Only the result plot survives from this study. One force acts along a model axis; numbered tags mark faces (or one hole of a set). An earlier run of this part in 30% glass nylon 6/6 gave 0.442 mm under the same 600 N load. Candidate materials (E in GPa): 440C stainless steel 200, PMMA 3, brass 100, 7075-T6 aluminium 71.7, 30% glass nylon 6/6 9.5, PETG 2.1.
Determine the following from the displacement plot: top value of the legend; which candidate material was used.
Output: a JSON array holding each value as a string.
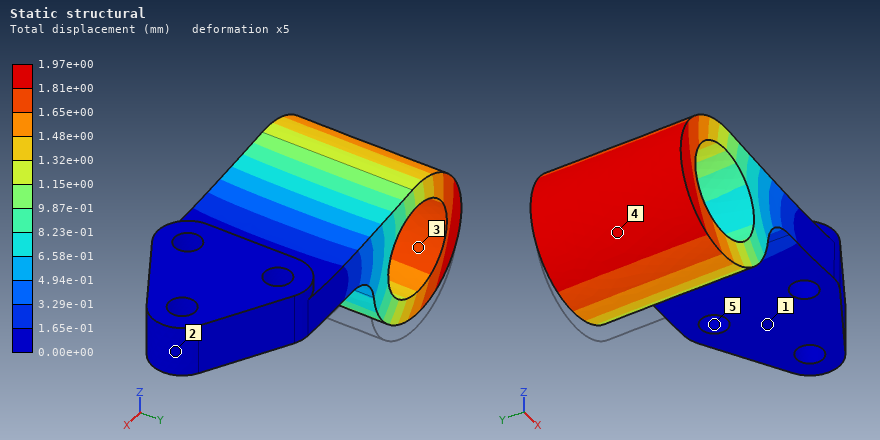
["1.97e+00 mm", "PETG"]
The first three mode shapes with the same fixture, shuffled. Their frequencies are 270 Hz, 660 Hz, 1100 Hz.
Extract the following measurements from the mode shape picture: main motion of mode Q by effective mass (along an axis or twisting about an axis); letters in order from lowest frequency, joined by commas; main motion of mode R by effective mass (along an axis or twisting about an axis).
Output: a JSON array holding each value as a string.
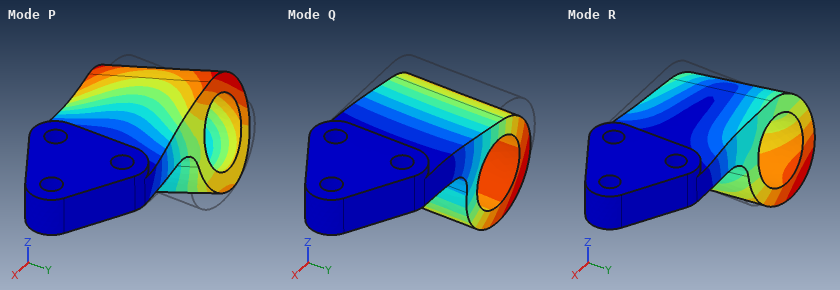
["along Z", "Q, R, P", "along Y"]
